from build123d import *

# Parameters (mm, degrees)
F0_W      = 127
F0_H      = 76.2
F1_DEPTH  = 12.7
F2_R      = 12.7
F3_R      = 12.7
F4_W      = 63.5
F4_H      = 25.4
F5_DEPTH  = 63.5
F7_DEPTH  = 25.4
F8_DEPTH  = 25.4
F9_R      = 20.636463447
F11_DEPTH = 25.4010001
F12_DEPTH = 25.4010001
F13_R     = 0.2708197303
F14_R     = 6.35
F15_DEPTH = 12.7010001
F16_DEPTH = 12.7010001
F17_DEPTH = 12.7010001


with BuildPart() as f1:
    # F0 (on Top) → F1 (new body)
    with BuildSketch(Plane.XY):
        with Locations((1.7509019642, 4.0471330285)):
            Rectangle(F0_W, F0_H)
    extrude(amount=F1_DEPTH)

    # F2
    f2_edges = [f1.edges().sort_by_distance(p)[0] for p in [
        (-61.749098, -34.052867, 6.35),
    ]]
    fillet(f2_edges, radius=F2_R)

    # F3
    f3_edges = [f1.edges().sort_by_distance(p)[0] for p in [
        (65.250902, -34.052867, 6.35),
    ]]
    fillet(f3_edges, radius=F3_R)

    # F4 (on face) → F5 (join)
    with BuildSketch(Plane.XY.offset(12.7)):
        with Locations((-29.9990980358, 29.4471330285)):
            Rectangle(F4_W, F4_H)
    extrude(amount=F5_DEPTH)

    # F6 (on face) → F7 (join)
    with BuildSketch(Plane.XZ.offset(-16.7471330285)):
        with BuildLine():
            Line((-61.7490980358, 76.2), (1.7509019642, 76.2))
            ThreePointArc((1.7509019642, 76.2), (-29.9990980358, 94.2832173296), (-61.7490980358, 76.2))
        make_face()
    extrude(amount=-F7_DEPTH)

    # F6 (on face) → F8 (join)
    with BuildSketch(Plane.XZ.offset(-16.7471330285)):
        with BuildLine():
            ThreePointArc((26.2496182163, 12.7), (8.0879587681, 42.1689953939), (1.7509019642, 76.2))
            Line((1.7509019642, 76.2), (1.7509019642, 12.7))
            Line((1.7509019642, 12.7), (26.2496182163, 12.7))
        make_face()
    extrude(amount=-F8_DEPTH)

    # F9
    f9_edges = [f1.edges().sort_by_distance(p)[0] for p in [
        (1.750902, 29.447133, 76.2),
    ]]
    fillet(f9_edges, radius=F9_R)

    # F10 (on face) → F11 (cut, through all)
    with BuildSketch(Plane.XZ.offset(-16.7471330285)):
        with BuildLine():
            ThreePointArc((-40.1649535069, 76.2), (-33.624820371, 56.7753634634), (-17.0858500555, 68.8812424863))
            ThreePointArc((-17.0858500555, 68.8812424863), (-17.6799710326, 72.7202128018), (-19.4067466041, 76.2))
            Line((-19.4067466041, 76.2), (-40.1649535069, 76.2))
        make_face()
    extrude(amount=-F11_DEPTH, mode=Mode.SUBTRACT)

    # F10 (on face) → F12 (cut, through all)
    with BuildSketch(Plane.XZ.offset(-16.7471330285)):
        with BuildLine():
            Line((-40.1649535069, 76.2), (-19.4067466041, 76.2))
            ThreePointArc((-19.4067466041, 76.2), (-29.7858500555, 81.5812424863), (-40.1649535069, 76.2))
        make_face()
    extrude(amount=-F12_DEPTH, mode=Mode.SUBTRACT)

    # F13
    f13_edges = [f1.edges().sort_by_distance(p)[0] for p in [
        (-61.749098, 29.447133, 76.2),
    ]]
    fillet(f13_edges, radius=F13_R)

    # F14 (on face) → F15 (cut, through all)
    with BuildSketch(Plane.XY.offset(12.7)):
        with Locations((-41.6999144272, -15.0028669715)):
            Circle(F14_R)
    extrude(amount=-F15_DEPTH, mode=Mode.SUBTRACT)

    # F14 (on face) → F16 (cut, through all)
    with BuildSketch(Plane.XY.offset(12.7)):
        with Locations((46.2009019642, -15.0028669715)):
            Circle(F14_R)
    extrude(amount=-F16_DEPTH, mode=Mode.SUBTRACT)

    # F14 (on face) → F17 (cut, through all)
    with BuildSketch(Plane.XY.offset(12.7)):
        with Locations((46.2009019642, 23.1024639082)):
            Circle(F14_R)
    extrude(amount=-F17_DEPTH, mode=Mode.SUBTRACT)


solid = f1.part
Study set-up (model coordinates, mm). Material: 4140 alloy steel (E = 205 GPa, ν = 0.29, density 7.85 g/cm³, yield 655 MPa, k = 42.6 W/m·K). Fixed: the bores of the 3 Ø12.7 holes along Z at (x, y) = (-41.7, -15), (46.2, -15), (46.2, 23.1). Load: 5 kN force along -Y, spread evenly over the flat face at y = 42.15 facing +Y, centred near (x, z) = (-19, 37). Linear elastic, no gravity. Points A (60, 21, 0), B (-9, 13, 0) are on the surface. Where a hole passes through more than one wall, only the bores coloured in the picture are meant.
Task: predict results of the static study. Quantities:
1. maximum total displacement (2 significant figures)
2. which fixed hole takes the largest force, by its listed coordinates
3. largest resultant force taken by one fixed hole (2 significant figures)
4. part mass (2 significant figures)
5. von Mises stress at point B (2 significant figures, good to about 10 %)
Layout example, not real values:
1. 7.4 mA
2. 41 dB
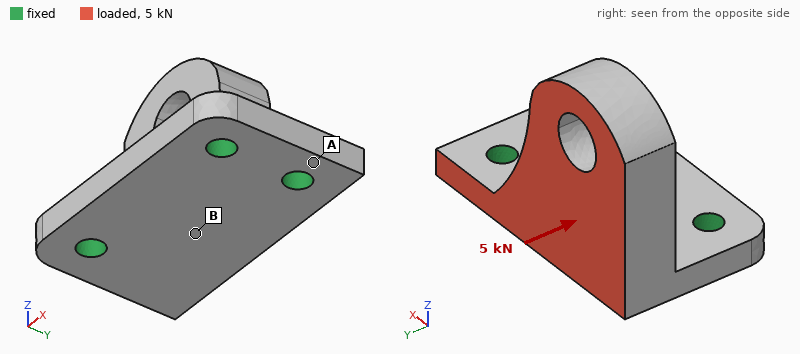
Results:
1. 100 µm
2. (-41.7, -15)
3. 3.2 kN
4. 1.9 kg
5. 32 MPa
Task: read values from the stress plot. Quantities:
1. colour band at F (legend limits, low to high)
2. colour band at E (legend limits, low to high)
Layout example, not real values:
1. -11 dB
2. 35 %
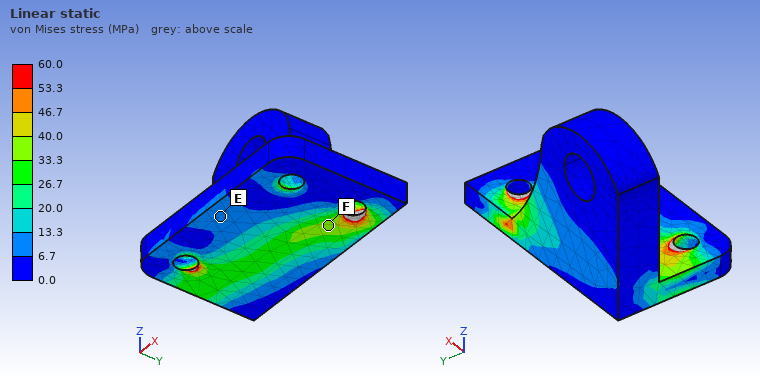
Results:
1. 33.3 to 40.0 MPa
2. 6.7 to 13.3 MPa
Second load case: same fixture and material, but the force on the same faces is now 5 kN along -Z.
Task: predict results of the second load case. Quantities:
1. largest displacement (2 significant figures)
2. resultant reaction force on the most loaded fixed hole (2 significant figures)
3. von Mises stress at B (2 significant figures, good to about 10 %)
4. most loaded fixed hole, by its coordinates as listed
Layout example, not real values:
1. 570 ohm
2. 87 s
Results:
1. 0.11 mm
2. 3.5 kN
3. 30 MPa
4. (46.2, 23.1)
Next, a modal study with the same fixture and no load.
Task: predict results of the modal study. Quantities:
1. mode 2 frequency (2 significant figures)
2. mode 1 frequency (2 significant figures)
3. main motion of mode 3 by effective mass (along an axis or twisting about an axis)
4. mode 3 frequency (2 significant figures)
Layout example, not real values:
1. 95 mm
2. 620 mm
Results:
1. 2700 Hz
2. 1100 Hz
3. along Z
4. 4500 Hz
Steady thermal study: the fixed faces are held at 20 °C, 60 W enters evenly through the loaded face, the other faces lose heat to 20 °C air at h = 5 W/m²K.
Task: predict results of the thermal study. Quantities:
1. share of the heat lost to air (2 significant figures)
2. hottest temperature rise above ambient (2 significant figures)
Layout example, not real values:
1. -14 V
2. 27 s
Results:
1. 7.0 %
2. 60 K
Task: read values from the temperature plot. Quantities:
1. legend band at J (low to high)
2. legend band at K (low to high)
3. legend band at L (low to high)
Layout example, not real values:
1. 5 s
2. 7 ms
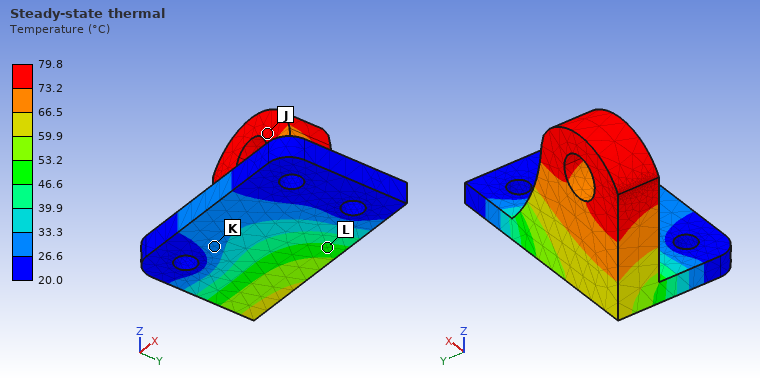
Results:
1. 73.2 to 79.8 °C
2. 26.6 to 33.3 °C
3. 46.6 to 53.2 °C
